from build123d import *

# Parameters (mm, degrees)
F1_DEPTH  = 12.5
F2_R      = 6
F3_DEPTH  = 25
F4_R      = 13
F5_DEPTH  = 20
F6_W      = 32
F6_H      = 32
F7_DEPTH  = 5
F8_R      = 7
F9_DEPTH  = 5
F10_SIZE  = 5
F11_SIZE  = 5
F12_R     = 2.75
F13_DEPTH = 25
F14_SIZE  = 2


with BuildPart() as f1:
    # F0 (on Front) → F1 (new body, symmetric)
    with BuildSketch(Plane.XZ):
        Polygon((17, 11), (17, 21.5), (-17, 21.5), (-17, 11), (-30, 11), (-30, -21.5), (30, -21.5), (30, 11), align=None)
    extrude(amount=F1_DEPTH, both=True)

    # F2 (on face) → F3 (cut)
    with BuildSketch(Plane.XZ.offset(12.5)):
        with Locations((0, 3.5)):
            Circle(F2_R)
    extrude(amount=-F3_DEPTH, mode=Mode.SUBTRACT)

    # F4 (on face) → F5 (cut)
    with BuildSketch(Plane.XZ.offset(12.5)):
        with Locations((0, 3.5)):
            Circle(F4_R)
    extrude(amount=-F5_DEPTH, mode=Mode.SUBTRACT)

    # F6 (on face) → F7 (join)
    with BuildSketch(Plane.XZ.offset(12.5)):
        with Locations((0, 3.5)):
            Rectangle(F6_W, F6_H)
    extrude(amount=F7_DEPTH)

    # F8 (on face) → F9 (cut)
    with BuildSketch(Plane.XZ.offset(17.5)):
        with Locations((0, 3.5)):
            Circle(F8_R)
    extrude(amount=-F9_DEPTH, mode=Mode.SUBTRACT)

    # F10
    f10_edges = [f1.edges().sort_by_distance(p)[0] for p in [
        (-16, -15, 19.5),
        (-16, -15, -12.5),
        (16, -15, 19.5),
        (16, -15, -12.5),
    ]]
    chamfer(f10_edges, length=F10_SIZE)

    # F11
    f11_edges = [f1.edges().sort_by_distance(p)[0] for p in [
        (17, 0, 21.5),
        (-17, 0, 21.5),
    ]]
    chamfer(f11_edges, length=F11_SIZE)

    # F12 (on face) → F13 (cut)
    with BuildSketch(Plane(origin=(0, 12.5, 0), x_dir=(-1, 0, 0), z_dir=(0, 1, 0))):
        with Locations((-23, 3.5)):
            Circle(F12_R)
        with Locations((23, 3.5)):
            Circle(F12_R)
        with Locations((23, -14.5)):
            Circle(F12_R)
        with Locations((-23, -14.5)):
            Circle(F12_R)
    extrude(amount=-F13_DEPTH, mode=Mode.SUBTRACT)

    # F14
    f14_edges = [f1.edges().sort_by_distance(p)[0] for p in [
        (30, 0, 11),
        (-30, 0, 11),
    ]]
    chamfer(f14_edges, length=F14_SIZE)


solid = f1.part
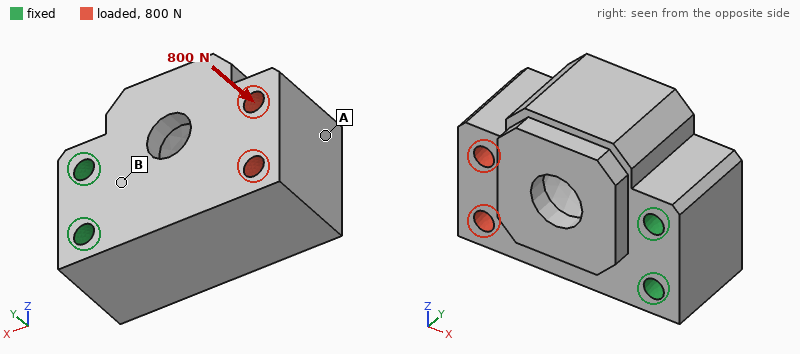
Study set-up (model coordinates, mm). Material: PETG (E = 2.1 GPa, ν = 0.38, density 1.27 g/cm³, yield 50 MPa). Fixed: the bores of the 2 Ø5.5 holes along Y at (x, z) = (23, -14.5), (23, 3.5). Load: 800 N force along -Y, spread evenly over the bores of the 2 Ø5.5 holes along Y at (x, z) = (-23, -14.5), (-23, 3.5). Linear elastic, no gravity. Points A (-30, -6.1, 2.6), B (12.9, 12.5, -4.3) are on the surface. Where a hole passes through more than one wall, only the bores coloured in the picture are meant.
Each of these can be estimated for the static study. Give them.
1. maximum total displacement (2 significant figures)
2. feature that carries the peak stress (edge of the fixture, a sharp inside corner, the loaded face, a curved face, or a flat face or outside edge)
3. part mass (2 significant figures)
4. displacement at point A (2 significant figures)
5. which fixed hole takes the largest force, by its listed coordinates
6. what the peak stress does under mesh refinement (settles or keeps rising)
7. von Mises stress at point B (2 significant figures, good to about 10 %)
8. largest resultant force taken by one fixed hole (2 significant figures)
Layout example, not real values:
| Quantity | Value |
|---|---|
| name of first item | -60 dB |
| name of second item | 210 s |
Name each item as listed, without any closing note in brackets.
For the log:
| Quantity | Value |
|---|---|
| maximum total displacement | 0.54 mm |
| feature that carries the peak stress | edge of the fixture |
| part mass | 60 g |
| displacement at point A | 0.53 mm |
| which fixed hole takes the largest force, by its listed coordinates | (23, -14.5) |
| what the peak stress does under mesh refinement | keeps rising |
| von Mises stress at point B | 8.4 MPa |
| largest resultant force taken by one fixed hole | 470 N |
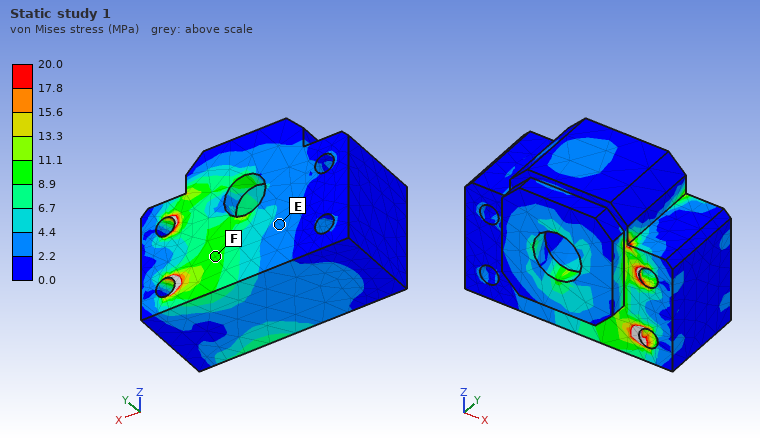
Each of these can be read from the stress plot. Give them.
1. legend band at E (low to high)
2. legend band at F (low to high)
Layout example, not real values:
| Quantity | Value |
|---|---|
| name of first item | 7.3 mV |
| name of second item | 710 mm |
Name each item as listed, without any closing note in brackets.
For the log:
| Quantity | Value |
|---|---|
| legend band at E | 2.2 to 4.4 MPa |
| legend band at F | 8.9 to 11.1 MPa |
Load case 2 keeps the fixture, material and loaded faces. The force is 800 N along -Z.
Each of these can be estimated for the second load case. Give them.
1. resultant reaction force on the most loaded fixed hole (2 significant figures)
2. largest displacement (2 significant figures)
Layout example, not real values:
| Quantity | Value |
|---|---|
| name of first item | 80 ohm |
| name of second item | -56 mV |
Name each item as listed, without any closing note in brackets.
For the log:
| Quantity | Value |
|---|---|
| resultant reaction force on the most loaded fixed hole | 1.7 kN |
| largest displacement | 0.45 mm |
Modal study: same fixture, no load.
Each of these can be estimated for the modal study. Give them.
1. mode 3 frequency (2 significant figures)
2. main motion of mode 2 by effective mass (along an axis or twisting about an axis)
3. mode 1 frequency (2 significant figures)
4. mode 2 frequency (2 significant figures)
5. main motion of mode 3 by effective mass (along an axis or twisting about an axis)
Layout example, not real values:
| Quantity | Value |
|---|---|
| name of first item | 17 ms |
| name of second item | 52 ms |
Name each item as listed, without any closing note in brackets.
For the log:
| Quantity | Value |
|---|---|
| mode 3 frequency | 2900 Hz |
| main motion of mode 2 by effective mass | along Z |
| mode 1 frequency | 1400 Hz |
| mode 2 frequency | 1500 Hz |
| main motion of mode 3 by effective mass | twisting about X |
